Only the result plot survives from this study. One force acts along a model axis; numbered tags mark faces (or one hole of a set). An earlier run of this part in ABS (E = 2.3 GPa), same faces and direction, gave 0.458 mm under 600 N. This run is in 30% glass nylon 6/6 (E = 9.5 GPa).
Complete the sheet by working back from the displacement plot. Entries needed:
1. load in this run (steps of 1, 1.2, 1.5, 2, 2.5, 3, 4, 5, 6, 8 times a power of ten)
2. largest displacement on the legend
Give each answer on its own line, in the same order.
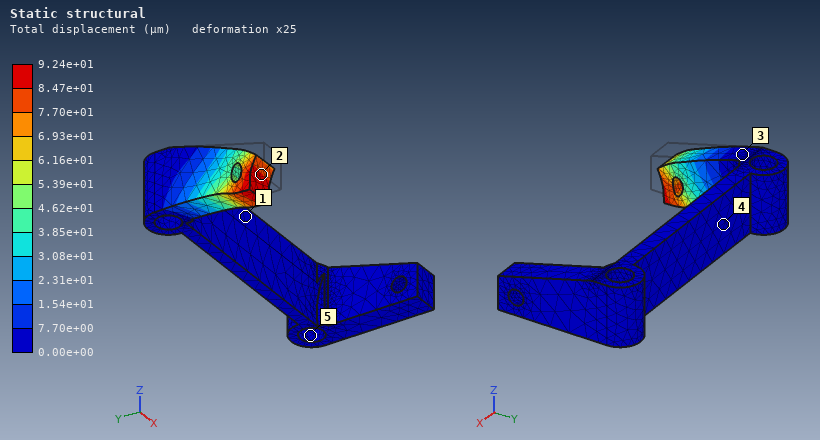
500 N
9.24e+01 µm
